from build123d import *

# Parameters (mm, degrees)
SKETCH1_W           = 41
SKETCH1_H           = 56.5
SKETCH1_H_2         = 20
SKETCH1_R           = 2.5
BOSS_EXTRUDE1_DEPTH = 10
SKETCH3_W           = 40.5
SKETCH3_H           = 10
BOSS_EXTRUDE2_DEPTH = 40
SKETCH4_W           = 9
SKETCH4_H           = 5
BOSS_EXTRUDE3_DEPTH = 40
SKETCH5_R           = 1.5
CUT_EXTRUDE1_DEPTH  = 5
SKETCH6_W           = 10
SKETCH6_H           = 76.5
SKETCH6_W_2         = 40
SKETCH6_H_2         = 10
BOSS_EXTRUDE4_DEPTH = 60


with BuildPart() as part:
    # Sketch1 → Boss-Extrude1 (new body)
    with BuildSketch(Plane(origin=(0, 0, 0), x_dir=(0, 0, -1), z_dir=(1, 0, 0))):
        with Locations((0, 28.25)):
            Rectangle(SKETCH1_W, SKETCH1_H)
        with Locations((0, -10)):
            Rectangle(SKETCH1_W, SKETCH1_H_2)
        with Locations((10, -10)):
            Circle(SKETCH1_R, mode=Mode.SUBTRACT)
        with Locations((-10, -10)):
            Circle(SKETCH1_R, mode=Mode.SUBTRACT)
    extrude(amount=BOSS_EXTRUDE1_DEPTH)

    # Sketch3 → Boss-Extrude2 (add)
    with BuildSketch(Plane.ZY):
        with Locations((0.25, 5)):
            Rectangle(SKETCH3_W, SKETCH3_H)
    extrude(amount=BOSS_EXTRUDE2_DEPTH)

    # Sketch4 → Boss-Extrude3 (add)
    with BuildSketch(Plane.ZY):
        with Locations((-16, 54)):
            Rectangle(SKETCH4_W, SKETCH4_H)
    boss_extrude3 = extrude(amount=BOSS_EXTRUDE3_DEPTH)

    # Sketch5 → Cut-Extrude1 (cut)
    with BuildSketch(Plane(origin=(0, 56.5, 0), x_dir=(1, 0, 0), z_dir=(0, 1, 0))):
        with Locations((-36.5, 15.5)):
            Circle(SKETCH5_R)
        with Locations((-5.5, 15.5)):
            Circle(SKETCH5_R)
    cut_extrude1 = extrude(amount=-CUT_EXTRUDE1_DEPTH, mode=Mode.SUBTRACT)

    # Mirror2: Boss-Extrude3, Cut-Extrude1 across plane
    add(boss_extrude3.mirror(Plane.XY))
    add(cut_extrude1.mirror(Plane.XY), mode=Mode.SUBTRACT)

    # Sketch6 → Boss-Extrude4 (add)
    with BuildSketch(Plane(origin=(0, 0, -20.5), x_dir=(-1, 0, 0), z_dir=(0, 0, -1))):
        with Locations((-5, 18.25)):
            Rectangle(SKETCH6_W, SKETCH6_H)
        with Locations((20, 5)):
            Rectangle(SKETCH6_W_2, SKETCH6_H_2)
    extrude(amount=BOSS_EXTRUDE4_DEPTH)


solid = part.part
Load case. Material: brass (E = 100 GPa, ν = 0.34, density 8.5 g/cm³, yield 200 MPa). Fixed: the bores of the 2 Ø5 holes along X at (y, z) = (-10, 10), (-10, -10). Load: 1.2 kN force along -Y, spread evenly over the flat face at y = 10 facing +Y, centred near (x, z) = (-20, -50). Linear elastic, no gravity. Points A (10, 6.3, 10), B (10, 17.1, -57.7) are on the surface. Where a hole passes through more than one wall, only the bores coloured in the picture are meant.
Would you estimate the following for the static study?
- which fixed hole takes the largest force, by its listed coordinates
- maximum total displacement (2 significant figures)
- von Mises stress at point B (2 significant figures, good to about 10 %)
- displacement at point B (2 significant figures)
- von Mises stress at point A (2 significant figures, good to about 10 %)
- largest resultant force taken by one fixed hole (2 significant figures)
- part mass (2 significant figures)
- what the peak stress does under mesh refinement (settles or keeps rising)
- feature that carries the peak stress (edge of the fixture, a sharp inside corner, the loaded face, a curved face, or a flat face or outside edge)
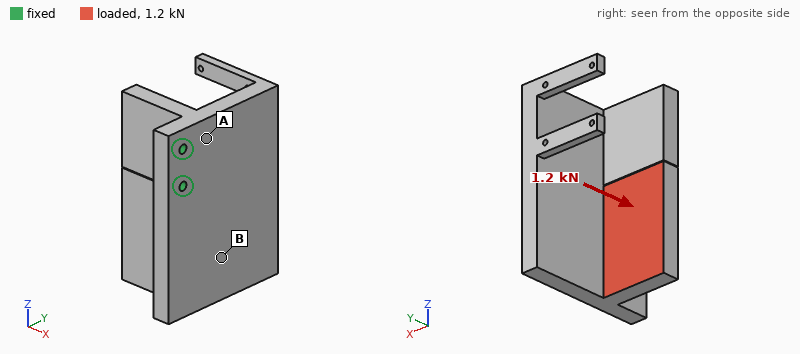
(-10, -10)
0.14 mm
8.1 MPa
0.046 mm
23 MPa
3.2 kN
1.0 kg
keeps rising
edge of the fixture
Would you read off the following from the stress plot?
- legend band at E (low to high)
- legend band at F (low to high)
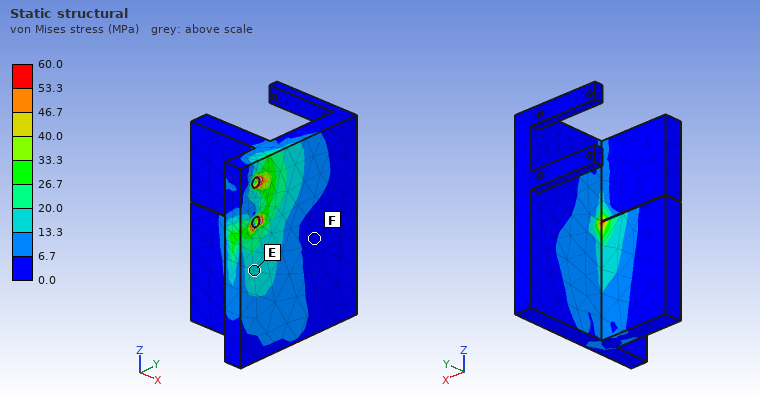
13.3 to 20.0 MPa
0.0 to 6.7 MPa
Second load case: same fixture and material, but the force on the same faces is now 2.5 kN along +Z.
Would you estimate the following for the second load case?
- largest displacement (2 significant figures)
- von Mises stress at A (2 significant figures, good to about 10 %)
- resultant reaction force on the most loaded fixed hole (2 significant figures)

0.24 mm
13 MPa
3.0 kN
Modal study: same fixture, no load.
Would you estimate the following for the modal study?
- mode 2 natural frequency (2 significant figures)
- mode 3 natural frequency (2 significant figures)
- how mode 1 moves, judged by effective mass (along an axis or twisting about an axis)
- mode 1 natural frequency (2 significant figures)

890 Hz
1400 Hz
along X
590 Hz
